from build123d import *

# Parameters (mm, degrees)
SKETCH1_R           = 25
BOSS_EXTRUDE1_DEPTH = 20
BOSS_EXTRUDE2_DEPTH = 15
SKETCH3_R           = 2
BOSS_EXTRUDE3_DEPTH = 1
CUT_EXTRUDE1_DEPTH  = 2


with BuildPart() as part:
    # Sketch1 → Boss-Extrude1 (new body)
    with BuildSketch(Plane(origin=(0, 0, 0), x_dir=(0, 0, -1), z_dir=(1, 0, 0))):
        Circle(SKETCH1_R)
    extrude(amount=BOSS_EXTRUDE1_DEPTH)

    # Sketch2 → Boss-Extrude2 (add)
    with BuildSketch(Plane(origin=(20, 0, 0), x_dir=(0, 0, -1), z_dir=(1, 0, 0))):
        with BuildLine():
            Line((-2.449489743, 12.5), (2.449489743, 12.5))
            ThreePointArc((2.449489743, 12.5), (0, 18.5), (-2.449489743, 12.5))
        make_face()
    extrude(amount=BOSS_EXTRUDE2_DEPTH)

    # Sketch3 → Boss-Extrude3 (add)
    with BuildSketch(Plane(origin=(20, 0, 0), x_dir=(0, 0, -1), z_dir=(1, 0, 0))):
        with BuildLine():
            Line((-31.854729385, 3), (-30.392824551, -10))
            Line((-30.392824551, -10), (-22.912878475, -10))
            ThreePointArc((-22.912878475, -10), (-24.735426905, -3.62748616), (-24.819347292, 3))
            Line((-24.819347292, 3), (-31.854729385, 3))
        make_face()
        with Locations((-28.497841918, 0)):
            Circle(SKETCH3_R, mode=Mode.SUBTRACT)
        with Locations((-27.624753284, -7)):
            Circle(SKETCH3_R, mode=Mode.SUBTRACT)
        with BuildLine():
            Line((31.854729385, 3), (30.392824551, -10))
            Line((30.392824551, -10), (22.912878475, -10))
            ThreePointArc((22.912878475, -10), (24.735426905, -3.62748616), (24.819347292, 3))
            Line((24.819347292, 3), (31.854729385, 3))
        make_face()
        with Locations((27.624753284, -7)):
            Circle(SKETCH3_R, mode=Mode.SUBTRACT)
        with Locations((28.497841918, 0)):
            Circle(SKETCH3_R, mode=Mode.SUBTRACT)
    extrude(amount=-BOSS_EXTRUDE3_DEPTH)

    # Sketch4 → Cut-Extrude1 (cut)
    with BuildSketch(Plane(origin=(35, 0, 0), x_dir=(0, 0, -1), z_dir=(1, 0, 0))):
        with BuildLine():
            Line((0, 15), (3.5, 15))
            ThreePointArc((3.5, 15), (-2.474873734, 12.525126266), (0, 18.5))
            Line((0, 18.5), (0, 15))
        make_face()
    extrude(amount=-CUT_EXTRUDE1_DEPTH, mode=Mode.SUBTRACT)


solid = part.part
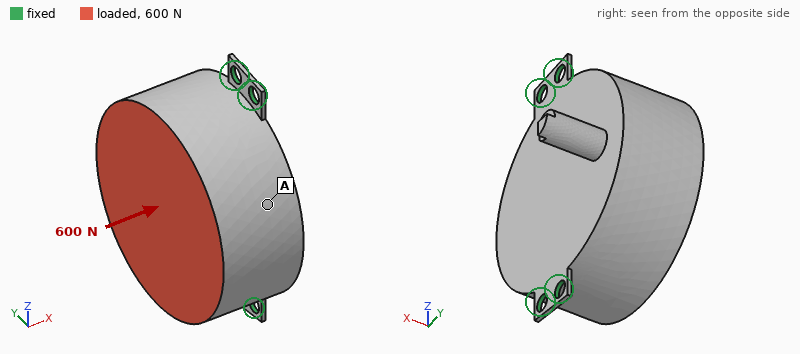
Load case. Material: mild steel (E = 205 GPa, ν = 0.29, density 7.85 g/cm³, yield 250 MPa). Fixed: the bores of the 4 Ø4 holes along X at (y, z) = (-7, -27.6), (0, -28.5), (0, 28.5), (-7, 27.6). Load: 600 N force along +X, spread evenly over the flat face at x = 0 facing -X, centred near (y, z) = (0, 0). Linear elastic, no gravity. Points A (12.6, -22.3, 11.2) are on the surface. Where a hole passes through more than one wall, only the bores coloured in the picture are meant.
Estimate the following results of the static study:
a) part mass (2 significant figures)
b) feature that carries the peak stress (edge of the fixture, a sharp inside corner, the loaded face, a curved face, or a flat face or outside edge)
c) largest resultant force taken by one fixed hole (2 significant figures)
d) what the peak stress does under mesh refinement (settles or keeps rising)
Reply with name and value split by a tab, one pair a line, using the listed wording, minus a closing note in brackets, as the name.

part mass	310 g
feature that carries the peak stress	edge of the fixture
largest resultant force taken by one fixed hole	320 N
what the peak stress does under mesh refinement	keeps rising
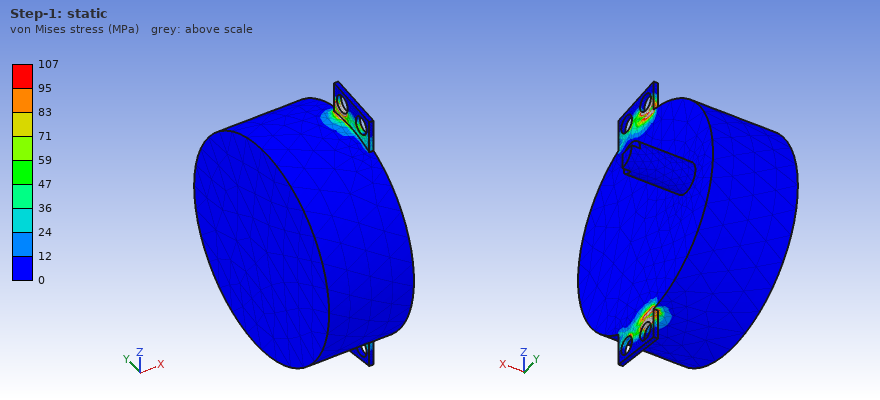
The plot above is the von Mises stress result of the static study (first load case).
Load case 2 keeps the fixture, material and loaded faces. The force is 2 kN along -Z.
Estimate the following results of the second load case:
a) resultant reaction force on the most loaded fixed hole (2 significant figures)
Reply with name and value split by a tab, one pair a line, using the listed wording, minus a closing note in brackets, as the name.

resultant reaction force on the most loaded fixed hole	640 N
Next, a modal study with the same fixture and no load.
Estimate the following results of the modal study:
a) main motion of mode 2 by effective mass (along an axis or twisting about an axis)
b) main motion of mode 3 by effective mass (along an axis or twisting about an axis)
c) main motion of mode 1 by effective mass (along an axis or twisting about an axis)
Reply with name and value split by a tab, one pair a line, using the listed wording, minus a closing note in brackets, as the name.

main motion of mode 2 by effective mass	along X
main motion of mode 3 by effective mass	along Z
main motion of mode 1 by effective mass	along Y
